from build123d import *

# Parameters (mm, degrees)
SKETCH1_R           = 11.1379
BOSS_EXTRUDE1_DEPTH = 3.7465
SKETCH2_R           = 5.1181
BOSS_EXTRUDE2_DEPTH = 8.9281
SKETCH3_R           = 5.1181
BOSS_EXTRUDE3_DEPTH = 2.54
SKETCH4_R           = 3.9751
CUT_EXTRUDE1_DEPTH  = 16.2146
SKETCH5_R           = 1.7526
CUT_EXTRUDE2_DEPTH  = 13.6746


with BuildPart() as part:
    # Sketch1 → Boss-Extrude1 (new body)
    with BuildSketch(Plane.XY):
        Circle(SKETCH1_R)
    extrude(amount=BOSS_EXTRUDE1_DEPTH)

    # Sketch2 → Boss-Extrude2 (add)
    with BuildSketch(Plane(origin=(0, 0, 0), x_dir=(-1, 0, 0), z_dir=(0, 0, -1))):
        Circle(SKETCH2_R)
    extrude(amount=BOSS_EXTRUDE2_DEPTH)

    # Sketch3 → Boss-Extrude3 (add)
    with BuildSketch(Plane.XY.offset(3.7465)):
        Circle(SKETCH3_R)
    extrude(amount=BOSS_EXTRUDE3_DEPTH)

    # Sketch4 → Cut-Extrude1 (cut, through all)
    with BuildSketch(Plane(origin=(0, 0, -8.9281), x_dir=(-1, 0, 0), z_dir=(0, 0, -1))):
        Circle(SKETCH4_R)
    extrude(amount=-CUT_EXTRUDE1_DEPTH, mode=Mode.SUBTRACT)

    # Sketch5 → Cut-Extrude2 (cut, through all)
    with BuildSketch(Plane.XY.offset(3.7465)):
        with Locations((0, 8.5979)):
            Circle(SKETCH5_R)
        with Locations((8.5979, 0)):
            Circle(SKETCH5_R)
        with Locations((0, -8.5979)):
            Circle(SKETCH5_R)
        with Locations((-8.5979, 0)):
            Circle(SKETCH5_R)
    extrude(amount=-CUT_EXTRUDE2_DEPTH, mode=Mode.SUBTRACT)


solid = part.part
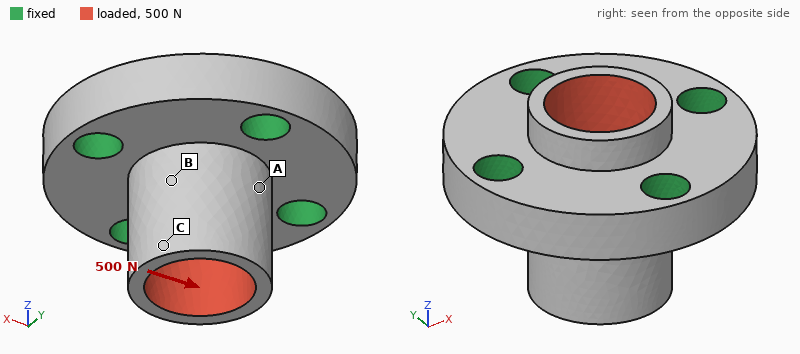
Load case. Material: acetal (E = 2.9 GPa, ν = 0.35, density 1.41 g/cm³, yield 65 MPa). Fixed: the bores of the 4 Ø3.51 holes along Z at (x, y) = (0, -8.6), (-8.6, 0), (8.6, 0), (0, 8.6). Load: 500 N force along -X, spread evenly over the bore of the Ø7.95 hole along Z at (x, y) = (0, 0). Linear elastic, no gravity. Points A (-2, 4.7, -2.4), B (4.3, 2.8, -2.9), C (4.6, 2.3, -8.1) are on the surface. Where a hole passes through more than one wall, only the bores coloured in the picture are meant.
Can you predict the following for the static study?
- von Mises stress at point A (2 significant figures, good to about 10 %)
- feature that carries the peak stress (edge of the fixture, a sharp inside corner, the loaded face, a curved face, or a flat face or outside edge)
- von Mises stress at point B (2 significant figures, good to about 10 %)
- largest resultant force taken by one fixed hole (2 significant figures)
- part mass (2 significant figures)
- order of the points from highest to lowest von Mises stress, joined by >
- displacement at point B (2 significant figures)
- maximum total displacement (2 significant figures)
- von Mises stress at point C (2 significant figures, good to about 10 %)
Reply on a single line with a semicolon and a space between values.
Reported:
16 MPa; a curved face; 10 MPa; 180 N; 2.1 g; A > B > C; 0.074 mm; 0.15 mm; 5.1 MPa
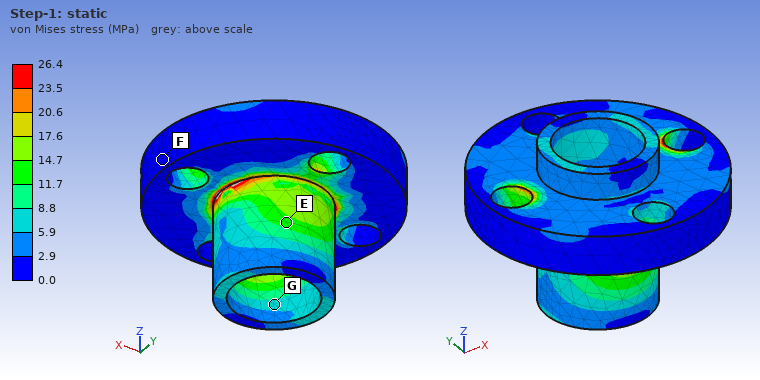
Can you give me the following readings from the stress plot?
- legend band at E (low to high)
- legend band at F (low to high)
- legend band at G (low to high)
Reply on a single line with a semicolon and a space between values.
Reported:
11.7 to 14.7 MPa; 0.0 to 2.9 MPa; 5.9 to 8.8 MPa
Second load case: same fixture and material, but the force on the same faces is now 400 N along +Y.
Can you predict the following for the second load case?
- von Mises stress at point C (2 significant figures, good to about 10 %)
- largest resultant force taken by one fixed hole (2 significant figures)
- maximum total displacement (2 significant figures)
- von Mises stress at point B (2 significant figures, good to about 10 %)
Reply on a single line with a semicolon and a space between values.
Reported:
2.7 MPa; 150 N; 0.12 mm; 12 MPa
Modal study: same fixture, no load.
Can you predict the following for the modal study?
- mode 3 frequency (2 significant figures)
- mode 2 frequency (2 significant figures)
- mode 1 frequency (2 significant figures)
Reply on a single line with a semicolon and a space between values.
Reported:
13 kHz; 13 kHz; 13 kHz
